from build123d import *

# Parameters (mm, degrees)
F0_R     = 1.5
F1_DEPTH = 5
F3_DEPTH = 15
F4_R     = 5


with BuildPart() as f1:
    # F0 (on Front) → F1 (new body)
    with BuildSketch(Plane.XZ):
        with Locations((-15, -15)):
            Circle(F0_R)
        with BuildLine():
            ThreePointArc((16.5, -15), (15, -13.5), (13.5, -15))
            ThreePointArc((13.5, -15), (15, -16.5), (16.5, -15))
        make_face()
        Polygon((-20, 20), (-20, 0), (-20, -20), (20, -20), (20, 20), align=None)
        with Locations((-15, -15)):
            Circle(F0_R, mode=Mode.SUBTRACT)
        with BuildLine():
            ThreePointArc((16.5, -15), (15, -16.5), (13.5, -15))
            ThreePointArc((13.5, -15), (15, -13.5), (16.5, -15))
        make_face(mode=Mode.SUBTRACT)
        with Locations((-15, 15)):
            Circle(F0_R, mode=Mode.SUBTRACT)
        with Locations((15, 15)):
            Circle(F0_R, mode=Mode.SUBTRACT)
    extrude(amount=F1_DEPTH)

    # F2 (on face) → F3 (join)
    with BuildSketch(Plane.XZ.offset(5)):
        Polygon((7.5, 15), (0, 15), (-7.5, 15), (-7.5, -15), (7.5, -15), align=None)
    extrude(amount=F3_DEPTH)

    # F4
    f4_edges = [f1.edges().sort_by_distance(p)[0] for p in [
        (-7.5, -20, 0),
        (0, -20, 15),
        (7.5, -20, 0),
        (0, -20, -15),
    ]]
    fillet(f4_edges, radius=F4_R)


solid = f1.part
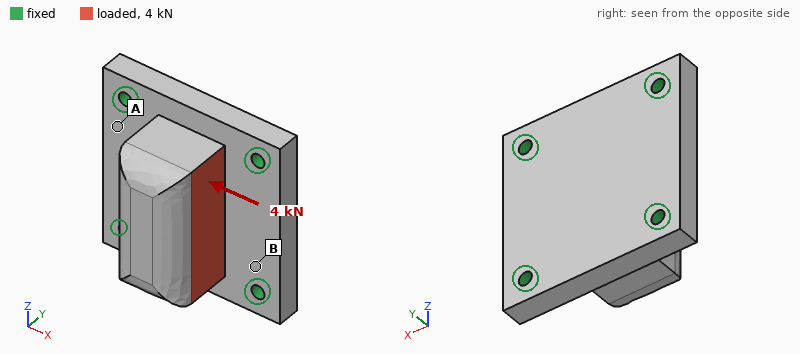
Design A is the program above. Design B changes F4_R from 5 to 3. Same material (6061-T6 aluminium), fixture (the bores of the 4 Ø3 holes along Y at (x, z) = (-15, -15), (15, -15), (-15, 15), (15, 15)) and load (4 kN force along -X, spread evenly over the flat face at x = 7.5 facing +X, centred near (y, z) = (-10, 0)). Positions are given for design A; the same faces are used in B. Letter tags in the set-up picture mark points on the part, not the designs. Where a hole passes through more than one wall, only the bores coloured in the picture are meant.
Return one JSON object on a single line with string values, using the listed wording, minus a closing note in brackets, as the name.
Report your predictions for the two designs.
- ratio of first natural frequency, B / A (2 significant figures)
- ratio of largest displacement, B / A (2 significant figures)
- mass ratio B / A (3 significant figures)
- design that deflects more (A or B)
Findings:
{"ratio of first natural frequency, B / A": "0.99", "ratio of largest displacement, B / A": "1.2", "mass ratio B / A": "1.02", "design that deflects more": "B"}
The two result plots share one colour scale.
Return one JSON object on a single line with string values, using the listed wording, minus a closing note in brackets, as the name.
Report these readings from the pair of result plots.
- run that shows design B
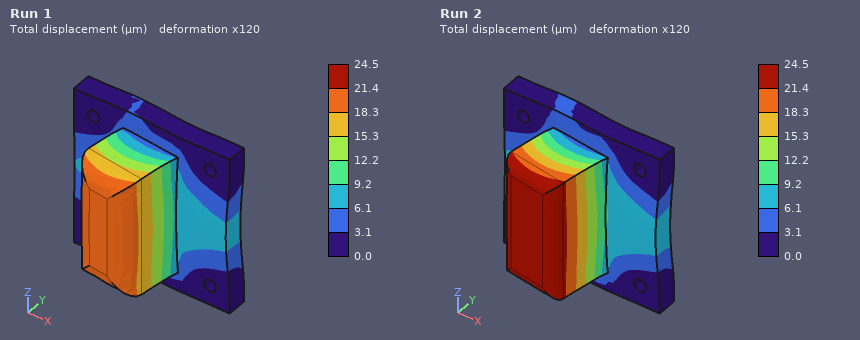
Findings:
{"run that shows design B": "Run 2"}
